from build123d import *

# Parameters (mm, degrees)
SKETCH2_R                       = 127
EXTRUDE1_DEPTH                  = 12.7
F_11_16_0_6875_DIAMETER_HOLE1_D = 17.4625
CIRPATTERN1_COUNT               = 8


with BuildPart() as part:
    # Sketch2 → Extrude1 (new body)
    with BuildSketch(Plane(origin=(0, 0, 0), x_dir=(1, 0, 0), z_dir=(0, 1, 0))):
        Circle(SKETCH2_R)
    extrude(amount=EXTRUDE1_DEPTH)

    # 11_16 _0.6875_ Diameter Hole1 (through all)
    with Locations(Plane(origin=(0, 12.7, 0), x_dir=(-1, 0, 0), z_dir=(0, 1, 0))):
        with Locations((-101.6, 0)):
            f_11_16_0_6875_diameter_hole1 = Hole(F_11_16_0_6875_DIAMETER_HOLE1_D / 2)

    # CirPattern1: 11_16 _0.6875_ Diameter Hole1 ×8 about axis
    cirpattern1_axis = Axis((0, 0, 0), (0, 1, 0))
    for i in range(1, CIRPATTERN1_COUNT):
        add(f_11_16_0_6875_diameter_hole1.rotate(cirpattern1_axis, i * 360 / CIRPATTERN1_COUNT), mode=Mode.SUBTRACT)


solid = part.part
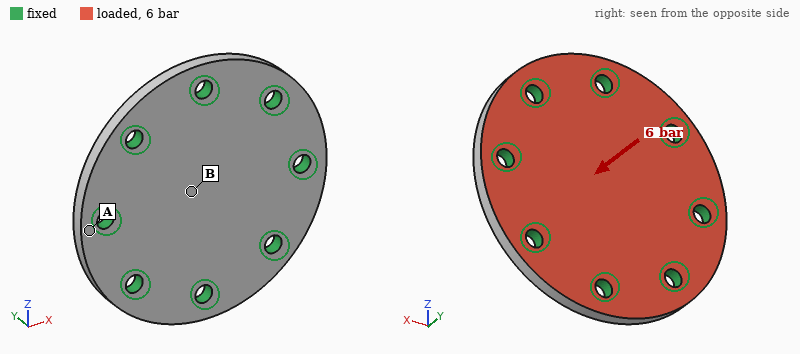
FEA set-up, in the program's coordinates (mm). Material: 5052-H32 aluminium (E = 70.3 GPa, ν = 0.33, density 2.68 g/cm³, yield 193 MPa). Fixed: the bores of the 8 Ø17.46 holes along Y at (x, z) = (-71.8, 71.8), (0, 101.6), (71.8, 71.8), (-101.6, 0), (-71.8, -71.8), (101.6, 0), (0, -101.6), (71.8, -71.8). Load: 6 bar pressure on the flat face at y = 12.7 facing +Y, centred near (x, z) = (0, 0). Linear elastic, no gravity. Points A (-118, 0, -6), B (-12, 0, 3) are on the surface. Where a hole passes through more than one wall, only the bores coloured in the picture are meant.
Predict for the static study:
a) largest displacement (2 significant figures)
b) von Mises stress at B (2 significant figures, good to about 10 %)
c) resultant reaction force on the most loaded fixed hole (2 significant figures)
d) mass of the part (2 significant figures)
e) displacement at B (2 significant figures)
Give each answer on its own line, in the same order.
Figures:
75 µm
18 MPa
3.7 kN
1.7 kg
73 µm
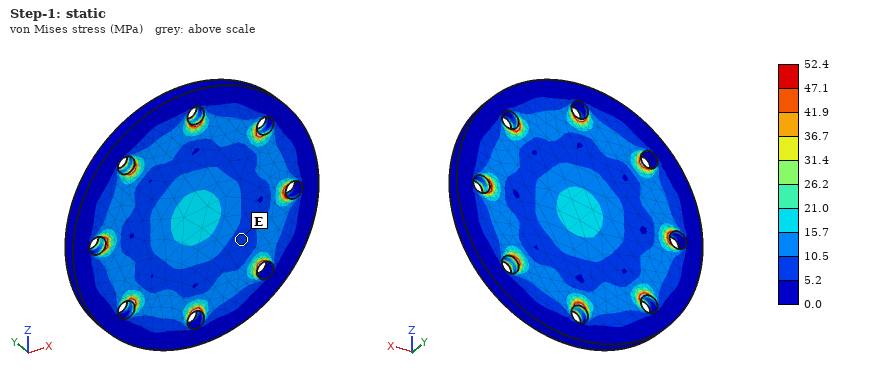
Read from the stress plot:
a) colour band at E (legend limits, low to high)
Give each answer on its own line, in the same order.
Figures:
5.2 to 10.5 MPa
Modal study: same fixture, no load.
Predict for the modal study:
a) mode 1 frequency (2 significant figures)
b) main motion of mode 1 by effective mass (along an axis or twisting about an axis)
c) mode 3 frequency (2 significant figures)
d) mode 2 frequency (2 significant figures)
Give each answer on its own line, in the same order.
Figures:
3000 Hz
along Y
6000 Hz
6000 Hz
